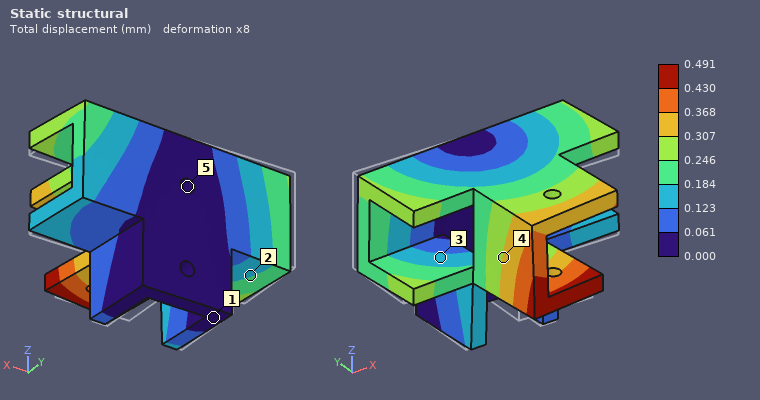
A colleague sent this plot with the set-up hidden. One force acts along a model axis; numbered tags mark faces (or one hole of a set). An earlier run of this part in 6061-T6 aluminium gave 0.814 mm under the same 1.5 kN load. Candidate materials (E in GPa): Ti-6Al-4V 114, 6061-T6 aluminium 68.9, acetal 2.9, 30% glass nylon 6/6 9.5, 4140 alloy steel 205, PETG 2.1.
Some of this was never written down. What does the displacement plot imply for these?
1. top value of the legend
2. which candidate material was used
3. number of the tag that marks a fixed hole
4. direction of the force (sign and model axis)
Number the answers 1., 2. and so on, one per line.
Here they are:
1. 0.491 mm
2. Ti-6Al-4V
3. 5
4. +X
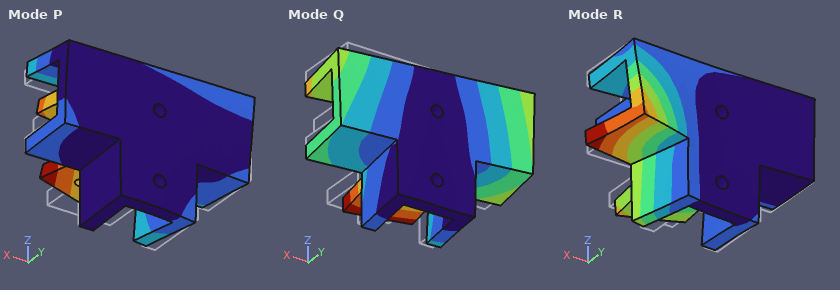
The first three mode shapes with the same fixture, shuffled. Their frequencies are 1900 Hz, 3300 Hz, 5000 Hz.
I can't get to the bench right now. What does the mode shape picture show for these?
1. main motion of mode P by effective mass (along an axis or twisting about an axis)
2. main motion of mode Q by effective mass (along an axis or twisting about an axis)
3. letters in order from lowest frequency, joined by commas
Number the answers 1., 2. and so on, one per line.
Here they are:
1. along Z
2. along X
3. Q, P, R
